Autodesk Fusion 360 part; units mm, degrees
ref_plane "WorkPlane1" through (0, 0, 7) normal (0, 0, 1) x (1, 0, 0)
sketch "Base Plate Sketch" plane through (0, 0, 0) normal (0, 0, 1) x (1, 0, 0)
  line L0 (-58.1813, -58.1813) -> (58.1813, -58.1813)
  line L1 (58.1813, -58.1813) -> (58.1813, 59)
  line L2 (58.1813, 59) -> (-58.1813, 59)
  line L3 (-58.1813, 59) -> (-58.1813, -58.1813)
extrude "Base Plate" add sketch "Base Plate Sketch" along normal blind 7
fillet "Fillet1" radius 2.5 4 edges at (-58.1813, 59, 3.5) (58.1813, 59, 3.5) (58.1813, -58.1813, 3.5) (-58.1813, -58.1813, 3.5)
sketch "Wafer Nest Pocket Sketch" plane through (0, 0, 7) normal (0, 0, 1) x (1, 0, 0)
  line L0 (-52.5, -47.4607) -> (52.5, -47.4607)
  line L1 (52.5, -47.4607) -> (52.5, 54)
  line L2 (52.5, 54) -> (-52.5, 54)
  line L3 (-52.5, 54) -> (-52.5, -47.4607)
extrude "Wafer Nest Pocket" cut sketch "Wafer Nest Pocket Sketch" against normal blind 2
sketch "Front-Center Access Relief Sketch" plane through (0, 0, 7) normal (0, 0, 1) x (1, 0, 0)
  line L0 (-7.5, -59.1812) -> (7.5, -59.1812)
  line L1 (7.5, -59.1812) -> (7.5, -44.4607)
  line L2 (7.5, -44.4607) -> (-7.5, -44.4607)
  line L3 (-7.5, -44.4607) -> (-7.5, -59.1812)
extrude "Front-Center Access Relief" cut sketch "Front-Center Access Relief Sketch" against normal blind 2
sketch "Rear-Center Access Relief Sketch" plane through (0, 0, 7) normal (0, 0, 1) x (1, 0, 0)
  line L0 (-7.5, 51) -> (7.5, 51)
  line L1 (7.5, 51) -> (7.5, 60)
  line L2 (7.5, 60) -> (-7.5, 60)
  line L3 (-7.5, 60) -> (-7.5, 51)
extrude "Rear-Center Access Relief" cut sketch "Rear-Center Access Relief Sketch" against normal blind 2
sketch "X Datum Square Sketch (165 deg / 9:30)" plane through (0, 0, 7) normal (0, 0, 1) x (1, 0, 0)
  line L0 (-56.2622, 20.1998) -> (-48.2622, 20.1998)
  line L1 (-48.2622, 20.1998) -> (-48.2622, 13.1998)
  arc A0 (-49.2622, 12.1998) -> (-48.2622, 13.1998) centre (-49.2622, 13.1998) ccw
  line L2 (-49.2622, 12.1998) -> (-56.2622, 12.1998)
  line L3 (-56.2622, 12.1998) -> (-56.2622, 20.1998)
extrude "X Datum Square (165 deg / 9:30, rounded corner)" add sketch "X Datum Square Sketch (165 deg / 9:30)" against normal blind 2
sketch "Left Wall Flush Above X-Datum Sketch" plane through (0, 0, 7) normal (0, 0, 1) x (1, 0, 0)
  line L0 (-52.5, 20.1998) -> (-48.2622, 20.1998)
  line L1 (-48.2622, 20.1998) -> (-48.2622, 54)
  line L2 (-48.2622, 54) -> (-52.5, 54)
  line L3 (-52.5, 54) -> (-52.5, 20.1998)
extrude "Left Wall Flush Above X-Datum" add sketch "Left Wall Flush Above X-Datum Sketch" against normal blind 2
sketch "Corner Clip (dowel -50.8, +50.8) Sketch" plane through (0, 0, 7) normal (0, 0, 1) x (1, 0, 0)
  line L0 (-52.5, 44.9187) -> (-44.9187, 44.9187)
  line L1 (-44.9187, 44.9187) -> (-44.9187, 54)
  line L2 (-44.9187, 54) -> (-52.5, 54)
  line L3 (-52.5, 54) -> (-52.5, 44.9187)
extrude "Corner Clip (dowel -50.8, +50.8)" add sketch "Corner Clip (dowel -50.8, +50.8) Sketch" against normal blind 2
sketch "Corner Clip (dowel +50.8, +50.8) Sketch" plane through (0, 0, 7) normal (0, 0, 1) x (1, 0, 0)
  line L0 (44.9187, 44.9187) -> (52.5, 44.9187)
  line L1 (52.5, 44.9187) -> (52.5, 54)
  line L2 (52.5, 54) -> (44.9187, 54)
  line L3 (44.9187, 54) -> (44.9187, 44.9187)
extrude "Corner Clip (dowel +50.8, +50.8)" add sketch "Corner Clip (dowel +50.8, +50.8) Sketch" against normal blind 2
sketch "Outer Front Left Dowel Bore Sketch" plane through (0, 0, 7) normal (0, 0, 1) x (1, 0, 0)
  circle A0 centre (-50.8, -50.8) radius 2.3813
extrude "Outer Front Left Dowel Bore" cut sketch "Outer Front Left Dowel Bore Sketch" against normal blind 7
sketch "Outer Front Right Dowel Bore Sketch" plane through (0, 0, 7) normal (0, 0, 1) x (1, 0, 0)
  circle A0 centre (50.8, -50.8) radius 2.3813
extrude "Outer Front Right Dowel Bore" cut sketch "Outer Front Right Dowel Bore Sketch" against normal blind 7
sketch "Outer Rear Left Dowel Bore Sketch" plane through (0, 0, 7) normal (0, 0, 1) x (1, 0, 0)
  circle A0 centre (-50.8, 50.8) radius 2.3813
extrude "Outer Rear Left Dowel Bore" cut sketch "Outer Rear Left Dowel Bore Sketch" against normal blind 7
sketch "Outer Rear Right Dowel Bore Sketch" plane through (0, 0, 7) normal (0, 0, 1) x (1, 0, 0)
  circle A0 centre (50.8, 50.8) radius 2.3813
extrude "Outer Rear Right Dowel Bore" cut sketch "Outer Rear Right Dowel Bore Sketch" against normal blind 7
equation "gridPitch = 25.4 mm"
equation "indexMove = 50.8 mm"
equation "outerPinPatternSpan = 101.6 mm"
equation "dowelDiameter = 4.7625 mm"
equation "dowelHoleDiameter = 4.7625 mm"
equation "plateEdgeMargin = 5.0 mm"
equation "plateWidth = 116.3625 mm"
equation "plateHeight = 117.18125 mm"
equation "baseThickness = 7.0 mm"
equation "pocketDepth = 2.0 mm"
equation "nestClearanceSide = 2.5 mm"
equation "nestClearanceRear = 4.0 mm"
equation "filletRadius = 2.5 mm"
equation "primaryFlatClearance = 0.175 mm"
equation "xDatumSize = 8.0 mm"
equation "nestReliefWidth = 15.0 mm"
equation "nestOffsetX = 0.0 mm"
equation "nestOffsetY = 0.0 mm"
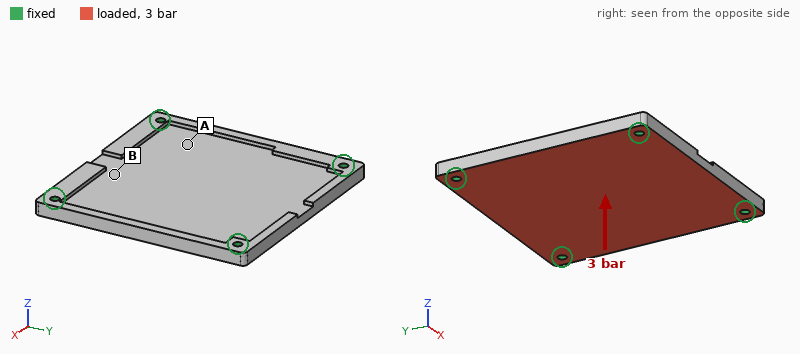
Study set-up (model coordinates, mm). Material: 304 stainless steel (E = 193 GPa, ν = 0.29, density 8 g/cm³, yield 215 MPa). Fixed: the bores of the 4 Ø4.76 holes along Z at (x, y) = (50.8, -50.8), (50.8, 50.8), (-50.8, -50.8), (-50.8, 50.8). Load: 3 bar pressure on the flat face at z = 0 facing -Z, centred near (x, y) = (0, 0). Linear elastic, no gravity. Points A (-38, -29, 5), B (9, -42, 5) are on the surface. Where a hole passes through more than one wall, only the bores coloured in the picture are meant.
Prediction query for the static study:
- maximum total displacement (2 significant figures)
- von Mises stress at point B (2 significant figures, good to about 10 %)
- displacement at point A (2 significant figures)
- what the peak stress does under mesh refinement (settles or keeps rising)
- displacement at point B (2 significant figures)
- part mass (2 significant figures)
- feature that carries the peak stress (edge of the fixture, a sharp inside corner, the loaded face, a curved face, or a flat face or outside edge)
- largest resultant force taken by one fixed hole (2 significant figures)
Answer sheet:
92 µm
27 MPa
38 µm
keeps rising
53 µm
590 g
edge of the fixture
1.2 kN
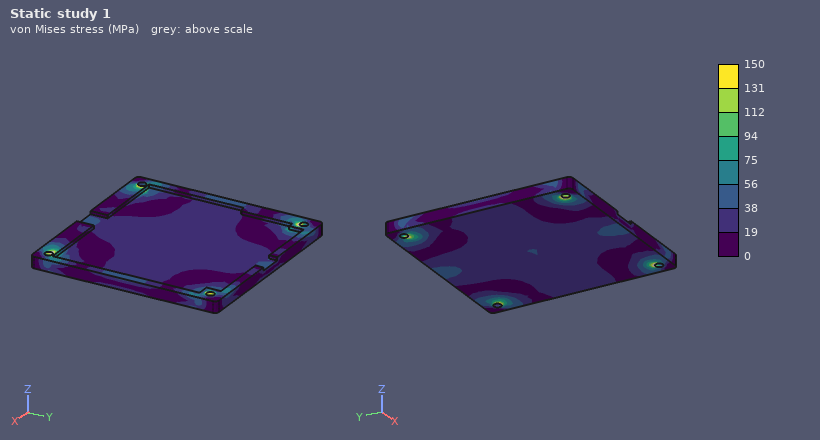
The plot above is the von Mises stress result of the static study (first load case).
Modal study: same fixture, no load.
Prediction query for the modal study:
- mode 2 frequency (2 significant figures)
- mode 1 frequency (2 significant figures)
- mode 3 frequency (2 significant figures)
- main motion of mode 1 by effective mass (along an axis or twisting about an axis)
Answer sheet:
3000 Hz
1800 Hz
3100 Hz
along Z
